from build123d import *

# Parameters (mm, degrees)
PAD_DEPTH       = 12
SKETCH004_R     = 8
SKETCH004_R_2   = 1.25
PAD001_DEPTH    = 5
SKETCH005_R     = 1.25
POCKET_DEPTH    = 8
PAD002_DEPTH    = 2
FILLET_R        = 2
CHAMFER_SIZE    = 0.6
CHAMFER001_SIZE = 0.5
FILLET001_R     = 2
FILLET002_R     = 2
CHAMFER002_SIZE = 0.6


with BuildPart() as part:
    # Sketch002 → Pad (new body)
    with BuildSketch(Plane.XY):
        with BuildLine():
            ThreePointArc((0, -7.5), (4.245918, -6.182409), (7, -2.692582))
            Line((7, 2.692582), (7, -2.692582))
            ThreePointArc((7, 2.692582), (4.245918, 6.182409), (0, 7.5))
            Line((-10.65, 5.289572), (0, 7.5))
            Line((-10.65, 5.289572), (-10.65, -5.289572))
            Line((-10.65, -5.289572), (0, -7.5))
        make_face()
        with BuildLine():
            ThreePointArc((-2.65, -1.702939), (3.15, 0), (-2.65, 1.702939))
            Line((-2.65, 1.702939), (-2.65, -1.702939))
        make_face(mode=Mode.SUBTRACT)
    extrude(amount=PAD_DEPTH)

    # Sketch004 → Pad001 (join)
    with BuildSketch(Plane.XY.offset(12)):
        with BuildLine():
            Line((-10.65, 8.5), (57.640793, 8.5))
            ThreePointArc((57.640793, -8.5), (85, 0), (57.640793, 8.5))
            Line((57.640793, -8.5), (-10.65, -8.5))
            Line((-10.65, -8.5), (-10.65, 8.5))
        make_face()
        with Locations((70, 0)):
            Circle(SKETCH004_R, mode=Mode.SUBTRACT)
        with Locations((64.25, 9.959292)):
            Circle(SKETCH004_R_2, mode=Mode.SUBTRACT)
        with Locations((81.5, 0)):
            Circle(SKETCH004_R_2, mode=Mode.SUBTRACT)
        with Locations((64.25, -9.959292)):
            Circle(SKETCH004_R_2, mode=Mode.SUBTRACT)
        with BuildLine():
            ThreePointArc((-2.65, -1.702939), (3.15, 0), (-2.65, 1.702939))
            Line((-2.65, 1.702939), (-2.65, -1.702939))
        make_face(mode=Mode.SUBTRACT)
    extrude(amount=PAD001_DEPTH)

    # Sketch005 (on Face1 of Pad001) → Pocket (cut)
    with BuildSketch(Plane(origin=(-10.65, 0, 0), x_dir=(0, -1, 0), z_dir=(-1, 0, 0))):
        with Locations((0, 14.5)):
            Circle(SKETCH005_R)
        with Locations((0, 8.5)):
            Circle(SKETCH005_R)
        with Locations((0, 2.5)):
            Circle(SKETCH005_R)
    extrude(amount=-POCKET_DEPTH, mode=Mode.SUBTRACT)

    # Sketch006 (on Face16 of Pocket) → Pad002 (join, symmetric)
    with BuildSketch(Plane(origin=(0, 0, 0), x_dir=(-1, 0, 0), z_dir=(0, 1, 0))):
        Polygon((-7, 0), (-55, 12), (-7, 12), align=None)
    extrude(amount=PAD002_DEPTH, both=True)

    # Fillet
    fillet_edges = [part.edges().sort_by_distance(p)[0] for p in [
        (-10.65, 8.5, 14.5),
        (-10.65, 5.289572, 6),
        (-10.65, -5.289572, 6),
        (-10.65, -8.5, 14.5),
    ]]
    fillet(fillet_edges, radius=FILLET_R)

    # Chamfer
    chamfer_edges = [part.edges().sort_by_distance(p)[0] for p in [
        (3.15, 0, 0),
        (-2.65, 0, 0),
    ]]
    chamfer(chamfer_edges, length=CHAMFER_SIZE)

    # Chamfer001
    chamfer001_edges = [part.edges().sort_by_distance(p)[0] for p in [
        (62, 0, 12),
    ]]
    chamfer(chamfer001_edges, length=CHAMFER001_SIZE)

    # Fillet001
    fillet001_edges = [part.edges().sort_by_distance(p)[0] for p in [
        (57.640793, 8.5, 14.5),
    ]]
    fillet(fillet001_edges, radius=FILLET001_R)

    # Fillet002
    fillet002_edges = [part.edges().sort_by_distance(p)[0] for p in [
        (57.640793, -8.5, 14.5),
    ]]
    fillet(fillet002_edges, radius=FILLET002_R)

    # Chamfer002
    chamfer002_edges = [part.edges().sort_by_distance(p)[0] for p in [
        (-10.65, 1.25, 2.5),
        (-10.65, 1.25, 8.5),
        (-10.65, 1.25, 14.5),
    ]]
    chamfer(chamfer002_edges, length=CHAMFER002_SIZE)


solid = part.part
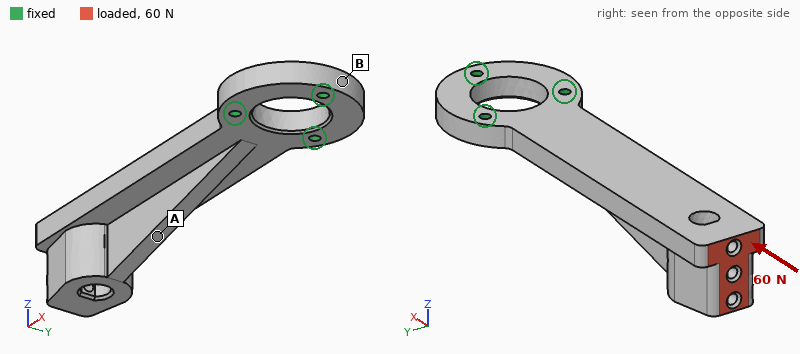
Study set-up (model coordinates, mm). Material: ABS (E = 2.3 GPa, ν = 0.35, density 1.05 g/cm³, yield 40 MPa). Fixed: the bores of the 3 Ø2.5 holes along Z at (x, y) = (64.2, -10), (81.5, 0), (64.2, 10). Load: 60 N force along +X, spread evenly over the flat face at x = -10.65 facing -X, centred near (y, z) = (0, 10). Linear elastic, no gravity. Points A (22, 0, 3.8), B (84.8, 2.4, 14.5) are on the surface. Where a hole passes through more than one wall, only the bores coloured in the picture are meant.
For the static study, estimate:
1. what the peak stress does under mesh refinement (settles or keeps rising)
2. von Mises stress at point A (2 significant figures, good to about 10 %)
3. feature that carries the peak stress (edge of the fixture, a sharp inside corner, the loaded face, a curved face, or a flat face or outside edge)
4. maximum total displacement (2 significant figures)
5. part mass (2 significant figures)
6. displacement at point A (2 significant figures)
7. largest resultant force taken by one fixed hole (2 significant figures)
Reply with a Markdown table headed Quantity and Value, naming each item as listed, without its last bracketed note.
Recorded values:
| Quantity | Value |
|---|---|
| what the peak stress does under mesh refinement | keeps rising |
| von Mises stress at point A | 1.5 MPa |
| feature that carries the peak stress | edge of the fixture |
| maximum total displacement | 1.1 mm |
| part mass | 12 g |
| displacement at point A | 0.56 mm |
| largest resultant force taken by one fixed hole | 34 N |
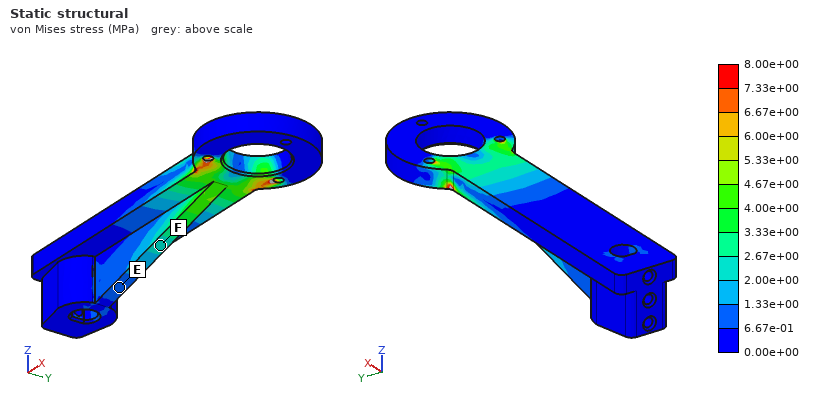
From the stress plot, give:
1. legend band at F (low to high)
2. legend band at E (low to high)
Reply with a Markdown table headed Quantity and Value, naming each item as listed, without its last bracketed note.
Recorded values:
| Quantity | Value |
|---|---|
| legend band at F | 2.00e+00 to 2.67e+00 MPa |
| legend band at E | 6.67e-01 to 1.33e+00 MPa |
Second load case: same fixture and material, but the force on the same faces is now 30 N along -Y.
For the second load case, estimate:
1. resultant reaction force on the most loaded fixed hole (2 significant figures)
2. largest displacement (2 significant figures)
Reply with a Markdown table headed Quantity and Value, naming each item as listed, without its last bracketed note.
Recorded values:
| Quantity | Value |
|---|---|
| resultant reaction force on the most loaded fixed hole | 120 N |
| largest displacement | 1.0 mm |
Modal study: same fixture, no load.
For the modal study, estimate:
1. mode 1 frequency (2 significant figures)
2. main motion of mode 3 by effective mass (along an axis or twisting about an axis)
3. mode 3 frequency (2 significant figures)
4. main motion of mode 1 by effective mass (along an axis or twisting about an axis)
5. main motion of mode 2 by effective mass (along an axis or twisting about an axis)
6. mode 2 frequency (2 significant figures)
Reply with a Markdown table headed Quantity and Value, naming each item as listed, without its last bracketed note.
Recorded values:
| Quantity | Value |
|---|---|
| mode 1 frequency | 160 Hz |
| main motion of mode 3 by effective mass | twisting about X |
| mode 3 frequency | 1200 Hz |
| main motion of mode 1 by effective mass | along Z |
| main motion of mode 2 by effective mass | along Y |
| mode 2 frequency | 480 Hz |
